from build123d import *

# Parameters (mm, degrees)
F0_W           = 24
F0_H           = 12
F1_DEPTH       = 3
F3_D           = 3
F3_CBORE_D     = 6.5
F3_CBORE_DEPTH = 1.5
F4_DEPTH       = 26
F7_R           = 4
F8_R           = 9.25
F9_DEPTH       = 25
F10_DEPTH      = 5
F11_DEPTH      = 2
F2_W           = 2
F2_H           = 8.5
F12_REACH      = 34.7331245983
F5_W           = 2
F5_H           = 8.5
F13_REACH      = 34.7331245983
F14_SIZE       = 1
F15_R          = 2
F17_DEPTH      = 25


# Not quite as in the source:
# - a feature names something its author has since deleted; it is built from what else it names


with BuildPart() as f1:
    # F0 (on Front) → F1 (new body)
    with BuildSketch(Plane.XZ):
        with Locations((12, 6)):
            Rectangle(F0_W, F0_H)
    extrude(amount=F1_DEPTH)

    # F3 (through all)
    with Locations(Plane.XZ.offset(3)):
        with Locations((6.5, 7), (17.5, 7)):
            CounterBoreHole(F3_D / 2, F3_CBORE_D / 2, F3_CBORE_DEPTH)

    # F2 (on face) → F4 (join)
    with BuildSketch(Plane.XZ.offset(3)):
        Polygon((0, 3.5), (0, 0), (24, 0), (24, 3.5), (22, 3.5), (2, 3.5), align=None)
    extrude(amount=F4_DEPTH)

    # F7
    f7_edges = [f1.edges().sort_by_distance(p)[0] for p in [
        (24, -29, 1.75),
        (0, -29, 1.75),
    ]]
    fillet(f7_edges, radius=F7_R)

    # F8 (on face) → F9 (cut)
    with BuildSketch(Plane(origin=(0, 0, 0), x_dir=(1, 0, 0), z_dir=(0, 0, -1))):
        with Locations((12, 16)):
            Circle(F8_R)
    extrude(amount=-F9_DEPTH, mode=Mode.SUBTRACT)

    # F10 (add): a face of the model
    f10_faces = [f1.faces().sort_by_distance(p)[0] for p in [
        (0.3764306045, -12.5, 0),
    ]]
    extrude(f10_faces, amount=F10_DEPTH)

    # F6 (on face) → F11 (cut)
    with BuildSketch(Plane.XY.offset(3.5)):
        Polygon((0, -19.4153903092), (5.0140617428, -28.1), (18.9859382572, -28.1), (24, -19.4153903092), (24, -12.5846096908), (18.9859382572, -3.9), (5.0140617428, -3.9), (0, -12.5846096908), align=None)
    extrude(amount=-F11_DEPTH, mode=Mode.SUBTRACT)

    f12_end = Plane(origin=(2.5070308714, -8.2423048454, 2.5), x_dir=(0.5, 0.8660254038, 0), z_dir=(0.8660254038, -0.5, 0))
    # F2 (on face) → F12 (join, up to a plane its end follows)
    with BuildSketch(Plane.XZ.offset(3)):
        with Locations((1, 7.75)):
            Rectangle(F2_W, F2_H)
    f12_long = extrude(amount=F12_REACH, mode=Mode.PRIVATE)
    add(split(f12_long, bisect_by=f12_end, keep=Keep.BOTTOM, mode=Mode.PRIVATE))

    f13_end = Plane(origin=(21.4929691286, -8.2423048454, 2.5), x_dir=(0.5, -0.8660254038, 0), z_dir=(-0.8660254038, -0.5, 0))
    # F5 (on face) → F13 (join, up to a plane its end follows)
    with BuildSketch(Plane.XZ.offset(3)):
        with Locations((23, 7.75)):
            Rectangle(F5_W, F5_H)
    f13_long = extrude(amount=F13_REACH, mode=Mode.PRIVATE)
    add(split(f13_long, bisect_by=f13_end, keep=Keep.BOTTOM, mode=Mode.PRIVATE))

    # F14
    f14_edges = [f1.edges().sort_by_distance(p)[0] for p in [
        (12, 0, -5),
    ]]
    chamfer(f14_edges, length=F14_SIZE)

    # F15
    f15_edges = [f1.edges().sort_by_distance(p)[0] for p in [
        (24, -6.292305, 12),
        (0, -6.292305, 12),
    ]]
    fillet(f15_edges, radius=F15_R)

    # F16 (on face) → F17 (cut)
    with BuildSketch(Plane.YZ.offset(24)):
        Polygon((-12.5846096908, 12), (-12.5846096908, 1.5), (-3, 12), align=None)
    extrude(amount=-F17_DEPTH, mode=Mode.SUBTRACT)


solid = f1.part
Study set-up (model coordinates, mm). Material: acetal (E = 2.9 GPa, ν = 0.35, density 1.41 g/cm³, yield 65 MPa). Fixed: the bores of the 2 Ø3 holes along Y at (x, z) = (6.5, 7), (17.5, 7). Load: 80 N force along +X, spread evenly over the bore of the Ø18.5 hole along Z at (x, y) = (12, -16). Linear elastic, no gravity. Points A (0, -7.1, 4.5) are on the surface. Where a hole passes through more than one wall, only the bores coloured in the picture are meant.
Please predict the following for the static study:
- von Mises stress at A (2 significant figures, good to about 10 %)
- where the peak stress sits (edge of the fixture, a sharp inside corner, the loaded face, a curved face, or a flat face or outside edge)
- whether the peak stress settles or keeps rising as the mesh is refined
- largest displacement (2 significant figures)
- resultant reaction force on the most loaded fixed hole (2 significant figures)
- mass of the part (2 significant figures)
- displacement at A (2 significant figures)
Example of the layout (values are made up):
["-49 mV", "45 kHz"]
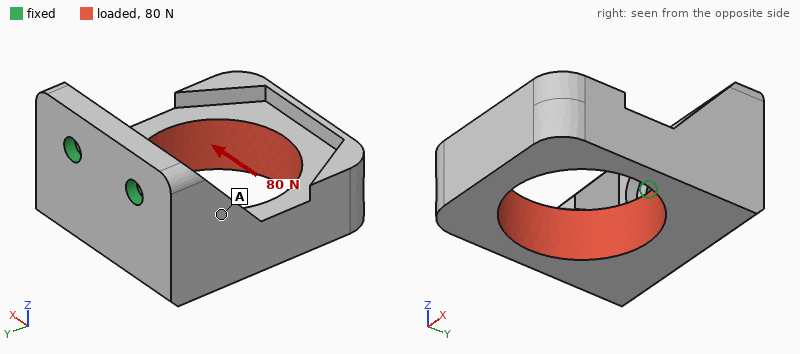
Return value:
["3.1 MPa", "edge of the fixture", "keeps rising", "0.49 mm", "110 N", "5.3 g", "0.14 mm"]
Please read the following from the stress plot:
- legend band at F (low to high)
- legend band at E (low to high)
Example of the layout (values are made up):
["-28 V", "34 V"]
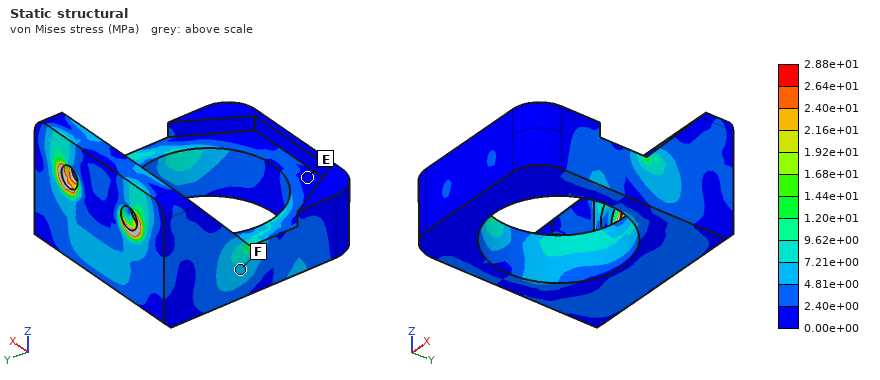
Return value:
["4.81e+00 to 7.21e+00 MPa", "0.00e+00 to 2.40e+00 MPa"]
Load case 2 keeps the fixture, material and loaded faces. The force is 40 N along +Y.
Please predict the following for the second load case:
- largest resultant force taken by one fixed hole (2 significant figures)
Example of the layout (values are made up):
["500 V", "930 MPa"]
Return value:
["20 N"]
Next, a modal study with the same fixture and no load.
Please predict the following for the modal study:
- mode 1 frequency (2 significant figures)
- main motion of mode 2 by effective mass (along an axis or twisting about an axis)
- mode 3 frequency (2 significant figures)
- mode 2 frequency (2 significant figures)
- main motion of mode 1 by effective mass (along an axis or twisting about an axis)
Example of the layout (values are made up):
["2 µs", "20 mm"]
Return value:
["620 Hz", "along X", "2700 Hz", "1200 Hz", "along Z"]
